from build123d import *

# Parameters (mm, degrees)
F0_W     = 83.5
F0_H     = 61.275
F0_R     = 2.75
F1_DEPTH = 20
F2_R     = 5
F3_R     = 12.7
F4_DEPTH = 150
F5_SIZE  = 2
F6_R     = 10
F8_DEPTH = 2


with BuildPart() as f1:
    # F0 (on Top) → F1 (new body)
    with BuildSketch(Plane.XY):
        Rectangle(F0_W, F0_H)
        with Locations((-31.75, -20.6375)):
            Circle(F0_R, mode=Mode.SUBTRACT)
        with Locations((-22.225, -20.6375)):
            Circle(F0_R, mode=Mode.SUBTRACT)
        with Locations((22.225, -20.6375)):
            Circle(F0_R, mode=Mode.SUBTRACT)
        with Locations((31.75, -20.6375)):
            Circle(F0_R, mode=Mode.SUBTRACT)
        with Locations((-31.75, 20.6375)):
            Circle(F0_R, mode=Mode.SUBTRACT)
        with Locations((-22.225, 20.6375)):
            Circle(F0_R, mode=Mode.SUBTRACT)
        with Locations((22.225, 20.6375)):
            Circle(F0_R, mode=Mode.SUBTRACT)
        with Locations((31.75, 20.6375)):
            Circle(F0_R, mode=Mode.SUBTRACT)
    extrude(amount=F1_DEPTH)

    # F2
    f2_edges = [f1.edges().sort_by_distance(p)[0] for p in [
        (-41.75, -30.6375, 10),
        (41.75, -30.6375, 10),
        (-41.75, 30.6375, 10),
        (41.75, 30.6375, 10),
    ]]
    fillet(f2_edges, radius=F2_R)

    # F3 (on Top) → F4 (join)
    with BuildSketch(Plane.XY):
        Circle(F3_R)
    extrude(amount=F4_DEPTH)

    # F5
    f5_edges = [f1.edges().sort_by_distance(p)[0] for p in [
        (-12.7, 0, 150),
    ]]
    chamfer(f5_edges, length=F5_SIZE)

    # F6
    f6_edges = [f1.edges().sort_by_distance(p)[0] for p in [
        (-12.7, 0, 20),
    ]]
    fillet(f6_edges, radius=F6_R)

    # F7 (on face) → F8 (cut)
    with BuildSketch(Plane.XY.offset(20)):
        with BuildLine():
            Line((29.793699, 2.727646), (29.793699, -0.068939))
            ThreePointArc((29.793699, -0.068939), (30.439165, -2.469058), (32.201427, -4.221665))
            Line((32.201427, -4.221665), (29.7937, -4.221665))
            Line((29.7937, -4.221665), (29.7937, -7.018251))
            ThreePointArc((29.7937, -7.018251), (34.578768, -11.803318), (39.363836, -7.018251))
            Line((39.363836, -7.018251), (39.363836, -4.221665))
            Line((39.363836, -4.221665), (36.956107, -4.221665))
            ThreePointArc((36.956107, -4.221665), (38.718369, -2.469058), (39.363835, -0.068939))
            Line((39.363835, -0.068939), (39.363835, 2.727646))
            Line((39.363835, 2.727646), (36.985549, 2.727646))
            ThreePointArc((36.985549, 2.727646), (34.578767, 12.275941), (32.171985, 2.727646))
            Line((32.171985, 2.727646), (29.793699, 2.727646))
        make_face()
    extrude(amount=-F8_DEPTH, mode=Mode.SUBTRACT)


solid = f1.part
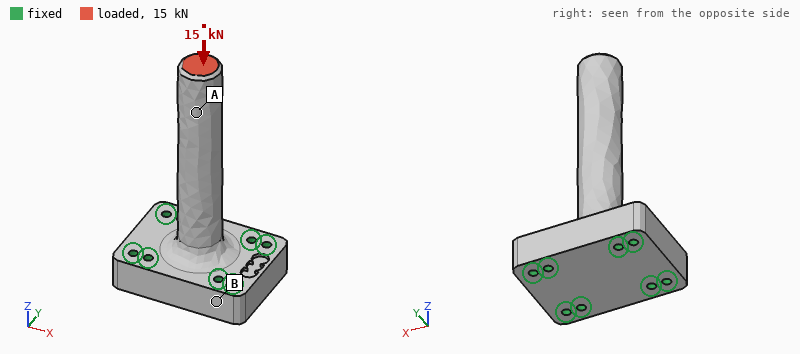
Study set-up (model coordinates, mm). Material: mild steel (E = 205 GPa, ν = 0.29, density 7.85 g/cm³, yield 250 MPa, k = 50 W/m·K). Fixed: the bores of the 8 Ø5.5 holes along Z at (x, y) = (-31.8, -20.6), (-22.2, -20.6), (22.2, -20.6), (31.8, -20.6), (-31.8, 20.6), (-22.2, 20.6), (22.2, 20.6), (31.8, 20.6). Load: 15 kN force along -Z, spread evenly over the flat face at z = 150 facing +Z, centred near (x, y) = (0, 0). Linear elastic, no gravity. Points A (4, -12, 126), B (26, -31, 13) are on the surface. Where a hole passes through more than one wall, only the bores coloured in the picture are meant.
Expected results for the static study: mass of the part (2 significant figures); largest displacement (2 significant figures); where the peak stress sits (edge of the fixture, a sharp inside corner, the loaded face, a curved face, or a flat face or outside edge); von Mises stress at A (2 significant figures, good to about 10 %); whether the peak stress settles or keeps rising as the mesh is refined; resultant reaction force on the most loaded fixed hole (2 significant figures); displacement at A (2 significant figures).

1.3 kg
22 µm
edge of the fixture
30 MPa
keeps rising
3.4 kN
18 µm
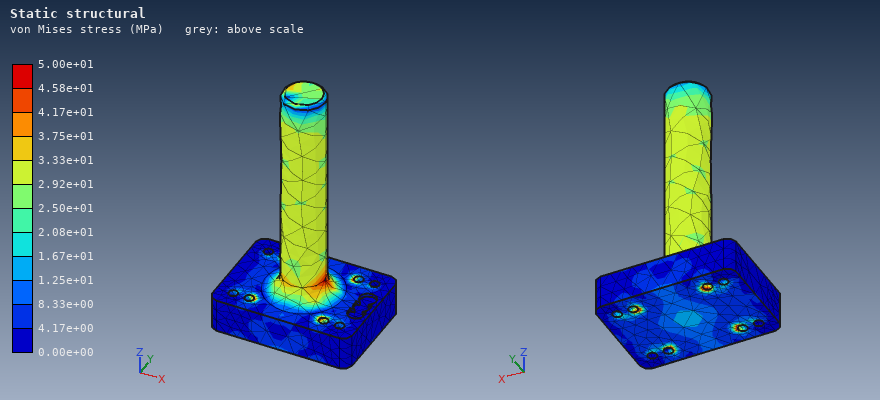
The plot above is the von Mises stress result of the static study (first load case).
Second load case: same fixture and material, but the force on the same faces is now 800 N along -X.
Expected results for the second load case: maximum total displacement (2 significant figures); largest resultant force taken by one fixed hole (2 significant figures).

0.14 mm
910 N
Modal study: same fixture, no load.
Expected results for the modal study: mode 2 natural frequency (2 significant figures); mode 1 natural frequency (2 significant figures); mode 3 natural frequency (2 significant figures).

1100 Hz
1000 Hz
5800 Hz
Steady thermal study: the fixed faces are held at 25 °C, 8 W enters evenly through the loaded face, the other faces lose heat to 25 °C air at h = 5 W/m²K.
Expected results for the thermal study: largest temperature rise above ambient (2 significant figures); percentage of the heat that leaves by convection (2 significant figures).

40 K
13 %
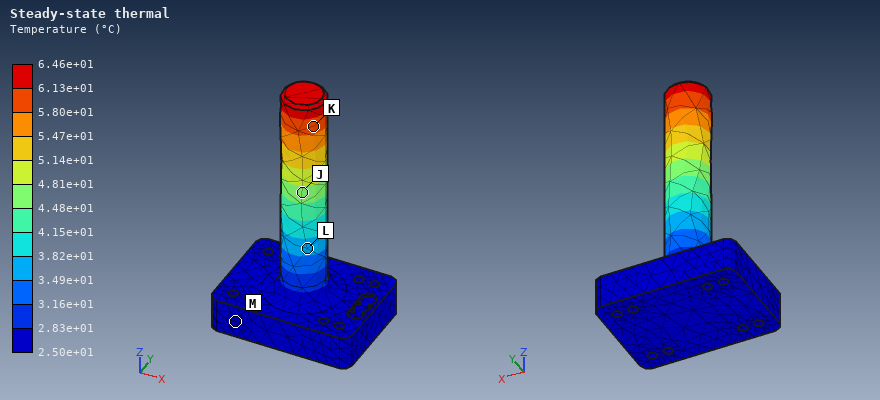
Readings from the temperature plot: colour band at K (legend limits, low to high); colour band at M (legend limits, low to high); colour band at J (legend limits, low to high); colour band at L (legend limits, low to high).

5.80e+01 to 6.13e+01 °C
2.50e+01 to 2.83e+01 °C
4.48e+01 to 4.81e+01 °C
3.49e+01 to 3.82e+01 °C
